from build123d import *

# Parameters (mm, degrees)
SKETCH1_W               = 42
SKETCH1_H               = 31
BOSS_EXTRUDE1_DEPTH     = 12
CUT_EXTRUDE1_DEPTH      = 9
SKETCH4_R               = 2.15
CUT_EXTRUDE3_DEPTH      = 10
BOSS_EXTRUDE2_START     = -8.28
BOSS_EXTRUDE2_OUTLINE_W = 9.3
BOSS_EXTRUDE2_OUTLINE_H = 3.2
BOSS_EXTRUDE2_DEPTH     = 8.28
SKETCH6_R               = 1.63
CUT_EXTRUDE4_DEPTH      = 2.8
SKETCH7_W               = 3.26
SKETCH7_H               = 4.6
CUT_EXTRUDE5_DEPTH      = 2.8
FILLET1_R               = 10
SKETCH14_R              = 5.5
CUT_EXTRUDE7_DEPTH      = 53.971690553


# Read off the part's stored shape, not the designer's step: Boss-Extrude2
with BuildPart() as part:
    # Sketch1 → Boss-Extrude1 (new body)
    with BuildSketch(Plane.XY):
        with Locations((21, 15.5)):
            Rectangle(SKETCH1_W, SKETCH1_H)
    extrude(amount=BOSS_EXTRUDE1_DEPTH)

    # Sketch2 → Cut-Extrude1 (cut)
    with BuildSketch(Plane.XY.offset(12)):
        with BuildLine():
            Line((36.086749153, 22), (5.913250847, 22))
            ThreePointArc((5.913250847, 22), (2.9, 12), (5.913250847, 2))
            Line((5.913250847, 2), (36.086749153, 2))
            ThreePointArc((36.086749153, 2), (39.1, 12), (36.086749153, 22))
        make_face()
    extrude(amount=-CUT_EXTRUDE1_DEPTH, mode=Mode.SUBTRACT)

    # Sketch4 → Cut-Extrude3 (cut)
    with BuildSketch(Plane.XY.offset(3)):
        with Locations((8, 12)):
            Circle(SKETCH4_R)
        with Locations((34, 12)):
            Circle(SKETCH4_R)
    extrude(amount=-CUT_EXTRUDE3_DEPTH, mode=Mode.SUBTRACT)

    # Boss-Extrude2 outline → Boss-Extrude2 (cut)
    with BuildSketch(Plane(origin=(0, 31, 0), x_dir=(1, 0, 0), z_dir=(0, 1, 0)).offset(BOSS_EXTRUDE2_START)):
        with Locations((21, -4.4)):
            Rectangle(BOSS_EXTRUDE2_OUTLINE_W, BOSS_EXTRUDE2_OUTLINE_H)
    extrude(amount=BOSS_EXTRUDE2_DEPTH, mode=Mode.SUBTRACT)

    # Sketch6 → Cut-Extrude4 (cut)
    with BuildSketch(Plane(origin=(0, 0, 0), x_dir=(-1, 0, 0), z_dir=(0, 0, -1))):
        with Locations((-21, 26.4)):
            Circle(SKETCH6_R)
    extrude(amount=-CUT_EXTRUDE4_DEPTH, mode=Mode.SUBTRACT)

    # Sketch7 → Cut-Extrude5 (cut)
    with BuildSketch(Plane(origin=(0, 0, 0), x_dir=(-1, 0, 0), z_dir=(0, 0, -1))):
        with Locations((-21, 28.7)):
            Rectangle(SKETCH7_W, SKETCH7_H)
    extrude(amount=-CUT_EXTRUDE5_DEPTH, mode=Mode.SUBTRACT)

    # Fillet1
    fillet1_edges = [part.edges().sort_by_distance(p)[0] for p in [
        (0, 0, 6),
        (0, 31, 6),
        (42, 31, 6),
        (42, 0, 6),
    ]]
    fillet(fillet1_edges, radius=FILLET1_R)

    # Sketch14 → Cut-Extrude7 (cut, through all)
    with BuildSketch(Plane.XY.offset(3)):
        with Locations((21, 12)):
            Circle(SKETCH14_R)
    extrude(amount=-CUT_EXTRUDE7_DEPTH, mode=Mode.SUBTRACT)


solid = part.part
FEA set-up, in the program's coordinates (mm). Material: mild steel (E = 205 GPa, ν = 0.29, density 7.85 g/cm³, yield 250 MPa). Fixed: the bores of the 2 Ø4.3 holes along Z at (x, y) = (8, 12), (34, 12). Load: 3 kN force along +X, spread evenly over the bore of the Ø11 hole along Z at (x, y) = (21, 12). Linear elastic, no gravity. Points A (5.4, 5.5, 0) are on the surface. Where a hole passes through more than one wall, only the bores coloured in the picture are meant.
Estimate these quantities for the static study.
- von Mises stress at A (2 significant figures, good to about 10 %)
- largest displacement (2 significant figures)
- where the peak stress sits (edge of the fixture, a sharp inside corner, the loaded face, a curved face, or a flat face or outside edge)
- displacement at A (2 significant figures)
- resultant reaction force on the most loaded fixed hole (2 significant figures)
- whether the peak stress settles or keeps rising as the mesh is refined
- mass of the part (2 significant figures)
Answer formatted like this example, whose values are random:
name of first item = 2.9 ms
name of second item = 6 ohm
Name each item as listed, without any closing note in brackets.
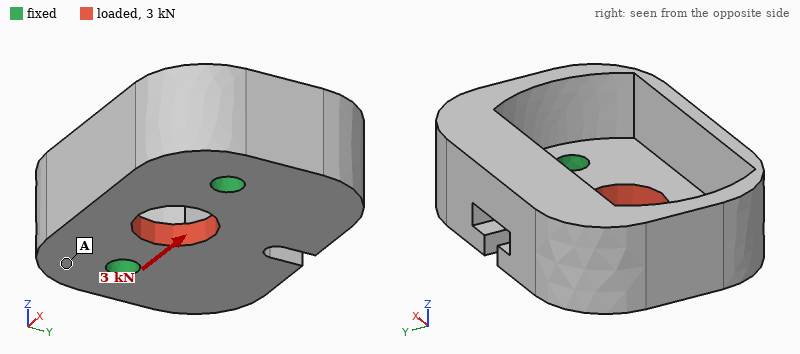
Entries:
von Mises stress at A = 11 MPa
largest displacement = 2.4 µm
where the peak stress sits = edge of the fixture
displacement at A = 0.80 µm
resultant reaction force on the most loaded fixed hole = 1.5 kN
whether the peak stress settles or keeps rising as the mesh is refined = keeps rising
mass of the part = 61 g
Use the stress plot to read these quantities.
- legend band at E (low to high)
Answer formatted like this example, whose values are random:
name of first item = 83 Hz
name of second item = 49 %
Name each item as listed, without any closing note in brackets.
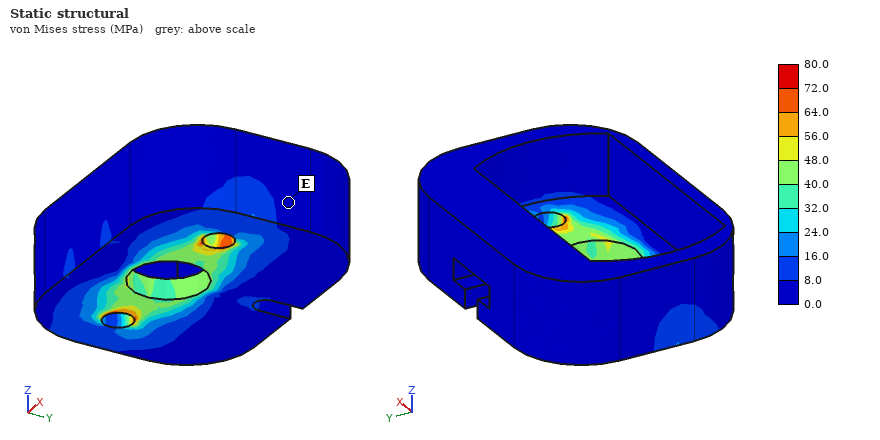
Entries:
legend band at E = 0.0 to 8.0 MPa
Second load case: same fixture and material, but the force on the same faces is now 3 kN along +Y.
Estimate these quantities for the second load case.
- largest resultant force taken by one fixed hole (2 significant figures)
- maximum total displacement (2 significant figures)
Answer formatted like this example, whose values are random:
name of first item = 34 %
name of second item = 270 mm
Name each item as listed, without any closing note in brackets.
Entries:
largest resultant force taken by one fixed hole = 1.5 kN
maximum total displacement = 4.1 µm
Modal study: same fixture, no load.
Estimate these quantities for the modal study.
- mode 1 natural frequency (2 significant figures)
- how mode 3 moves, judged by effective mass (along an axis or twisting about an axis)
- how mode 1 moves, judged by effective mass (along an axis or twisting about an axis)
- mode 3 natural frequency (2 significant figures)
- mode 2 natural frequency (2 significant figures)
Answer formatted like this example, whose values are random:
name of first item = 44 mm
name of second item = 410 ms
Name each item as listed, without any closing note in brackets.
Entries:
mode 1 natural frequency = 5100 Hz
how mode 3 moves, judged by effective mass = along Z
how mode 1 moves, judged by effective mass = along Z
mode 3 natural frequency = 14 kHz
mode 2 natural frequency = 10 kHz
